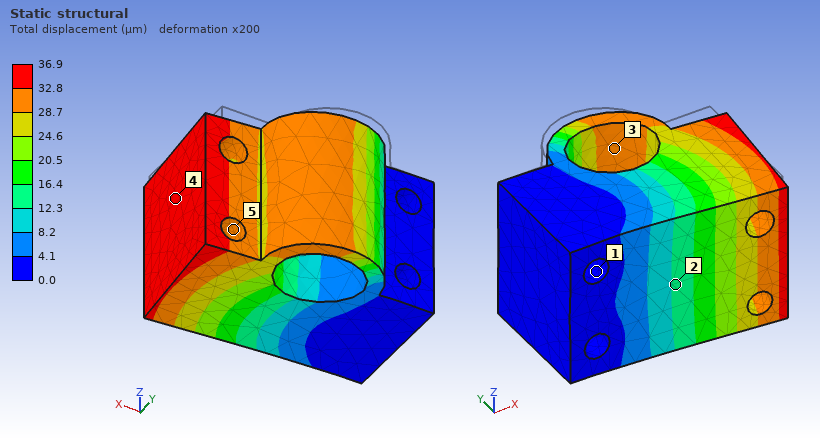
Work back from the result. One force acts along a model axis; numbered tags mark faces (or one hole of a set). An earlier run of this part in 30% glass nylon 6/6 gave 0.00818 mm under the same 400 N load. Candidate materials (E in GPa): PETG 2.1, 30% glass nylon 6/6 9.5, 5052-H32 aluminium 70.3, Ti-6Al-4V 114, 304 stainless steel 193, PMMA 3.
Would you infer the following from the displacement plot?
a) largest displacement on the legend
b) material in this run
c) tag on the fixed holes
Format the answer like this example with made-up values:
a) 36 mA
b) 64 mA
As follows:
a) 36.9 µm
b) PETG
c) 1
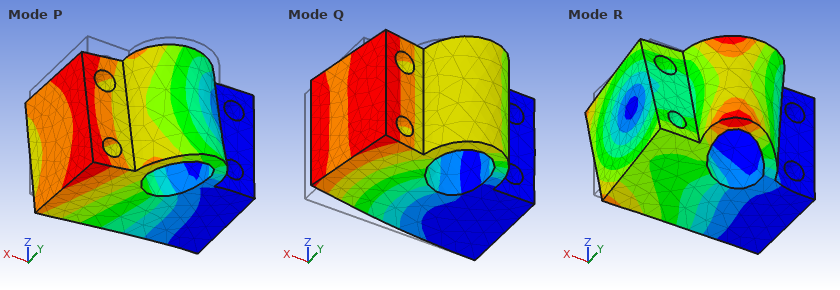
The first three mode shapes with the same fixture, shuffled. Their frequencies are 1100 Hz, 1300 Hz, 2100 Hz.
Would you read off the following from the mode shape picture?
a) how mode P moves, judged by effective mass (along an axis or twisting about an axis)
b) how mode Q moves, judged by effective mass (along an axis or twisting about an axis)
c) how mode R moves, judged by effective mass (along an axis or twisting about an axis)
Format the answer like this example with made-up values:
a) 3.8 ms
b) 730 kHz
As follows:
a) along Z
b) along Y
c) twisting about X
